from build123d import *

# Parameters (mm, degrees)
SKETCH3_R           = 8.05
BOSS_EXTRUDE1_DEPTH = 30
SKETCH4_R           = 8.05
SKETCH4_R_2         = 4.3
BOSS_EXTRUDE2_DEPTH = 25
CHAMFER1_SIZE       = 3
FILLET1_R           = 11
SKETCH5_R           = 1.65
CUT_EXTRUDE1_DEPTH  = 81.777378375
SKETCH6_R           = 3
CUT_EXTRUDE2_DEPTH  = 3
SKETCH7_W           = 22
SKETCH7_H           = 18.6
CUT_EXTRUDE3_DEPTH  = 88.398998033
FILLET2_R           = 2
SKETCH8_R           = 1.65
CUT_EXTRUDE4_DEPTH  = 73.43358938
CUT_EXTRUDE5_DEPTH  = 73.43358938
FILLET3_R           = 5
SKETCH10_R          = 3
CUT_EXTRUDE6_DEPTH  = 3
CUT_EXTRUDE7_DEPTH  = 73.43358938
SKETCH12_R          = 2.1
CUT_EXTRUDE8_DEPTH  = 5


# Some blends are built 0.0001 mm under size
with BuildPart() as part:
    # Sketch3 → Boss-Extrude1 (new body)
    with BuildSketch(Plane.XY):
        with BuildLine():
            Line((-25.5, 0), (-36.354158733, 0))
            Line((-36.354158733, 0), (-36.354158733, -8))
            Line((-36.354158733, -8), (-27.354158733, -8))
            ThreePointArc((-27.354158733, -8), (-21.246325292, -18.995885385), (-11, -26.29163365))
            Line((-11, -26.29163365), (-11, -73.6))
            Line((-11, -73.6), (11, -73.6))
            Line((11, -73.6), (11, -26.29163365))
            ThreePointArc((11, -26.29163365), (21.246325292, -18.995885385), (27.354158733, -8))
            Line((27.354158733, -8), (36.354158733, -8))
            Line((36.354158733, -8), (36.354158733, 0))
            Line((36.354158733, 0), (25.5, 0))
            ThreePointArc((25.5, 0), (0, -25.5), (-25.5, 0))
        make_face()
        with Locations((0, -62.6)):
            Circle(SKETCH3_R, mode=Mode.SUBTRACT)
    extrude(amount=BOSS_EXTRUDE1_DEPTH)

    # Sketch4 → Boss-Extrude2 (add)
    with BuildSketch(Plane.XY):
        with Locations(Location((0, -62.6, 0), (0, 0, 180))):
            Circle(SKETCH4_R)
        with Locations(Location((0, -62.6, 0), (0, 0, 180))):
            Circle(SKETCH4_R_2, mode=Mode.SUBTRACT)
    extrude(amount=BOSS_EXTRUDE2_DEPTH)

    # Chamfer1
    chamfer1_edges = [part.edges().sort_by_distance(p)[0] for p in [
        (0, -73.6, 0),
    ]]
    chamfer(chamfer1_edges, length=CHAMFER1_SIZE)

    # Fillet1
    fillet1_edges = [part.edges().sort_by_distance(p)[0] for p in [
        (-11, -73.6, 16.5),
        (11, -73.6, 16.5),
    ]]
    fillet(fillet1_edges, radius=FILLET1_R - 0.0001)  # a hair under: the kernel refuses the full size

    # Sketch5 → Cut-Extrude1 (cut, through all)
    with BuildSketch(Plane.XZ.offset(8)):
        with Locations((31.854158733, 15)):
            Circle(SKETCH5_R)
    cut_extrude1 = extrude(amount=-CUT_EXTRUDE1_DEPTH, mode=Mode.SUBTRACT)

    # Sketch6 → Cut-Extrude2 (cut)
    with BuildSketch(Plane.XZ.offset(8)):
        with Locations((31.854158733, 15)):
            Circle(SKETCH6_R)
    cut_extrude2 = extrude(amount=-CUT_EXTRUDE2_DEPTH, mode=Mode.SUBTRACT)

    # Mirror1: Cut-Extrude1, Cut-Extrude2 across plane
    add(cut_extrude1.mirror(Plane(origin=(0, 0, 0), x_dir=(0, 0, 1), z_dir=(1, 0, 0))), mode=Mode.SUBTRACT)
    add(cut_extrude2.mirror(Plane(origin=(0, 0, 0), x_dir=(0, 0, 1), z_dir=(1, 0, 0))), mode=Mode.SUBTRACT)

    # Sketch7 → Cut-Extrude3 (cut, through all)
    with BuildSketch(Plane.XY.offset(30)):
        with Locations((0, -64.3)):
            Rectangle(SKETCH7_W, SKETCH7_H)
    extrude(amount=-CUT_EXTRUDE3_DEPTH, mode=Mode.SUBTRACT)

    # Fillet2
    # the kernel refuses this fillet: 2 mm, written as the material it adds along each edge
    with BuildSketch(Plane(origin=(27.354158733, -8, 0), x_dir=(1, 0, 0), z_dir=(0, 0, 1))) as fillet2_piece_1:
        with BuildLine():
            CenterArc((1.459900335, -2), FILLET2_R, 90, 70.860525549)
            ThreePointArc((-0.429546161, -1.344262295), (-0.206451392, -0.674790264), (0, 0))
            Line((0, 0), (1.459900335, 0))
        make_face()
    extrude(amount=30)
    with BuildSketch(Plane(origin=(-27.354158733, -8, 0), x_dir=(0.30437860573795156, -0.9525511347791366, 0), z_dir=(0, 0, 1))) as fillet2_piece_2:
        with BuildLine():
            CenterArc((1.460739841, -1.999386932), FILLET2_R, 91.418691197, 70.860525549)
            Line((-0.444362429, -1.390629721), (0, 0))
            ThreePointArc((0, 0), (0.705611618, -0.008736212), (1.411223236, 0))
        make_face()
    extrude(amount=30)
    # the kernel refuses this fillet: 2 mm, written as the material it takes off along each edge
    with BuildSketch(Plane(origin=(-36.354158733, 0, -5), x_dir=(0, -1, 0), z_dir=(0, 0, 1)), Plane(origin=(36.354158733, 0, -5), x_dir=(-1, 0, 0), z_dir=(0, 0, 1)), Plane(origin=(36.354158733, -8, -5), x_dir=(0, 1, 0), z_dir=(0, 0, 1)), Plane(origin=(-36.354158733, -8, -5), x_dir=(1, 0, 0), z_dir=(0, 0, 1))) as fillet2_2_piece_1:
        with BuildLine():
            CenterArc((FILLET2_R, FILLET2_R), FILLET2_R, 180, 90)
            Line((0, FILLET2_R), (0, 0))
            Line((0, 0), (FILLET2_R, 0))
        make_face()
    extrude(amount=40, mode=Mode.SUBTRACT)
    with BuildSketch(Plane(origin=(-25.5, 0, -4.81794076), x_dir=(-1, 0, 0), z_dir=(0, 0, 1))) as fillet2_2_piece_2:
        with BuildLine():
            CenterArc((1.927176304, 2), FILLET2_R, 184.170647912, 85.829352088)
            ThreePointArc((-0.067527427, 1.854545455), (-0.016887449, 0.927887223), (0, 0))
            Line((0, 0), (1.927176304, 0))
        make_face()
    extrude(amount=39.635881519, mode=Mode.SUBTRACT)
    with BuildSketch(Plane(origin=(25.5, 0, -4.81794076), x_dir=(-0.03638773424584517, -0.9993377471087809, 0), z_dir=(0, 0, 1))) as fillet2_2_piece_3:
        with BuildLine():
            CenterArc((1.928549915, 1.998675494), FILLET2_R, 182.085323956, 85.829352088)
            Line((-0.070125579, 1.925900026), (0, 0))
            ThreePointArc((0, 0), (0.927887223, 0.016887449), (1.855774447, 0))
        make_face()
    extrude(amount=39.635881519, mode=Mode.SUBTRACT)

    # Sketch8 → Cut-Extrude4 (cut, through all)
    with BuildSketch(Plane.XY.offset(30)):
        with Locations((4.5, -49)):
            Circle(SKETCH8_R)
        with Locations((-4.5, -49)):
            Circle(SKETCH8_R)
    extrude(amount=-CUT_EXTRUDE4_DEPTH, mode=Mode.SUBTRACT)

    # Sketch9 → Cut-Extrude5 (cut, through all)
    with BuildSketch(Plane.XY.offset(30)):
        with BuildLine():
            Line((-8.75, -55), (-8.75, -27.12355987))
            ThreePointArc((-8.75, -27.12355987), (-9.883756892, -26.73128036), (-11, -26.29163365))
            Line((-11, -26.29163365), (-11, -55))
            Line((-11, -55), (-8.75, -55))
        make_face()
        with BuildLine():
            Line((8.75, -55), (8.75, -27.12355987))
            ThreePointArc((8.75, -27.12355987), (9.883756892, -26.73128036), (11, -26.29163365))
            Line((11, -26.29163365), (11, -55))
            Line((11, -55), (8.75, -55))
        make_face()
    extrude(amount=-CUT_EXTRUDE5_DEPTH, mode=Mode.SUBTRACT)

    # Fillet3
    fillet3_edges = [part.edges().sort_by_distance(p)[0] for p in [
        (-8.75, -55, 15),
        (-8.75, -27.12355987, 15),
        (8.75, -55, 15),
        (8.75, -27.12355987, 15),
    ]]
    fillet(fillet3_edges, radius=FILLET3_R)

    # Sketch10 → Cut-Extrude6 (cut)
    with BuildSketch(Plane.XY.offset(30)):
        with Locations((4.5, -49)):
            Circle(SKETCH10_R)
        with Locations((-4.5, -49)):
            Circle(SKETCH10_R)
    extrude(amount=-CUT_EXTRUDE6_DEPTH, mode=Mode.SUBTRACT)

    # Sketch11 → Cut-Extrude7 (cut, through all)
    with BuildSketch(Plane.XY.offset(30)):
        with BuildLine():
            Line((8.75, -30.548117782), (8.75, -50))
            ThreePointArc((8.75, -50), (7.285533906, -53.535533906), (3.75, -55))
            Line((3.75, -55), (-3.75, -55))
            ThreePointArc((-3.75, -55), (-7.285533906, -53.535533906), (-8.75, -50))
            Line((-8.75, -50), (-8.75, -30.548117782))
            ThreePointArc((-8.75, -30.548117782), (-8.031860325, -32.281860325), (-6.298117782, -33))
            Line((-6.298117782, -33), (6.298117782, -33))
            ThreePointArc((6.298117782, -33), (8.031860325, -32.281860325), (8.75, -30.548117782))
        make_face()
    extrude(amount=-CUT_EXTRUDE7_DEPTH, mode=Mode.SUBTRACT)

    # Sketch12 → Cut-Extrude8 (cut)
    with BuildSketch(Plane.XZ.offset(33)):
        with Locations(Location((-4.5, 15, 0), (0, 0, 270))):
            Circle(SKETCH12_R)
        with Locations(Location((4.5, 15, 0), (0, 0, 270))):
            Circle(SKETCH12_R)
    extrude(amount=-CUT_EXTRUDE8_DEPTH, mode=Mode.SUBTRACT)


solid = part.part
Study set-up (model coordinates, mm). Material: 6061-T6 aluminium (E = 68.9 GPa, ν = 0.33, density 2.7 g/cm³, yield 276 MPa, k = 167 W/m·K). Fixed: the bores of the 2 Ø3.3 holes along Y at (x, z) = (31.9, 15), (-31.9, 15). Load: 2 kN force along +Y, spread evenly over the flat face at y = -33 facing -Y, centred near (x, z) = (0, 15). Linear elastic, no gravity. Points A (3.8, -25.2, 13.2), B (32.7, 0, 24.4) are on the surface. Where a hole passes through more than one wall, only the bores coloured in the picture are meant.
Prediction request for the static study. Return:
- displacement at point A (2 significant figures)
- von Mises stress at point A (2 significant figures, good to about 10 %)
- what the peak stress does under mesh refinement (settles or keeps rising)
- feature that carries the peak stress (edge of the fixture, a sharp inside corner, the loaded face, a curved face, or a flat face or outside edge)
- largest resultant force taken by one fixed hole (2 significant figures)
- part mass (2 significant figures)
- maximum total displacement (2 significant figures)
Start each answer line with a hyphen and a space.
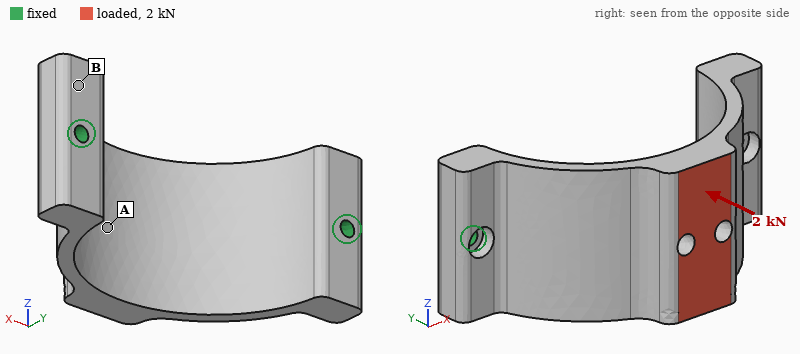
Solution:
- 26 µm
- 15 MPa
- keeps rising
- edge of the fixture
- 1.3 kN
- 37 g
- 29 µm
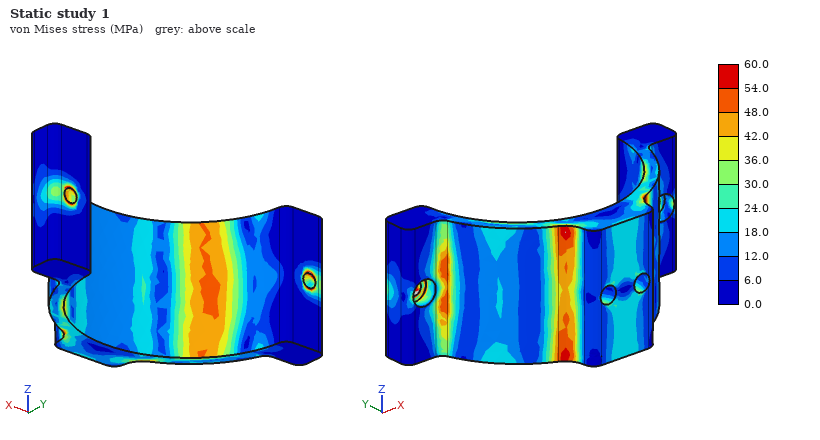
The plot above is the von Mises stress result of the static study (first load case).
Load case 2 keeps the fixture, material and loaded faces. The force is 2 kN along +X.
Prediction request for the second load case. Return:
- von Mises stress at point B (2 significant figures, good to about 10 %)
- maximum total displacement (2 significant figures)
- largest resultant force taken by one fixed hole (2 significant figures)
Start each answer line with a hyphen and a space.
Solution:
- 9.0 MPa
- 62 µm
- 1.3 kN
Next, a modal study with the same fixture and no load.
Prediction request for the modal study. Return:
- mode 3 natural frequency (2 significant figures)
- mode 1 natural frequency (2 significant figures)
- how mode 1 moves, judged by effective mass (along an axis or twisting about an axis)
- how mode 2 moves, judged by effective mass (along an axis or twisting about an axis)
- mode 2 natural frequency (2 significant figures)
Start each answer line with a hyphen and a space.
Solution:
- 9800 Hz
- 3100 Hz
- along Z
- along X
- 5100 Hz
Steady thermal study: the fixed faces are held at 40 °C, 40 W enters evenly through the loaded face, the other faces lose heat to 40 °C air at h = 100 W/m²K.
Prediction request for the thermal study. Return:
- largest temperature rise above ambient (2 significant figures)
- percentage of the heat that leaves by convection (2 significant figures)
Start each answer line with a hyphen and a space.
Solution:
- 40 K
- 31 %
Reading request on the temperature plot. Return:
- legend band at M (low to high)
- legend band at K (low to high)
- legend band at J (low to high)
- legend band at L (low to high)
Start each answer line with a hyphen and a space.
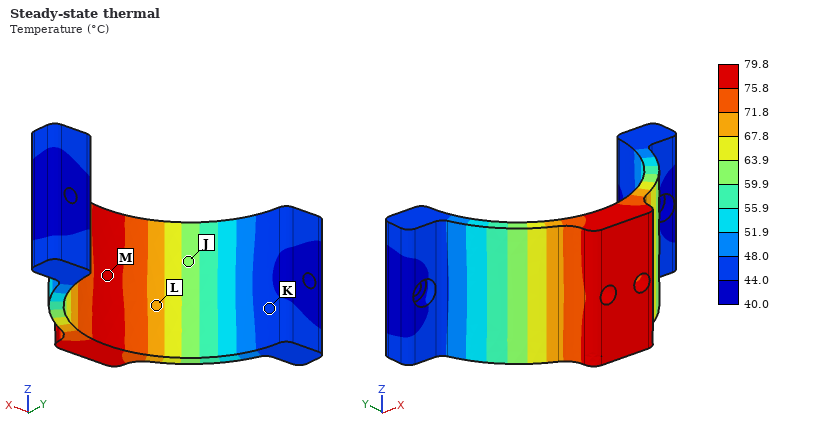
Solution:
- 75.8 to 79.8 °C
- 44.0 to 48.0 °C
- 59.9 to 63.9 °C
- 67.8 to 71.8 °C
